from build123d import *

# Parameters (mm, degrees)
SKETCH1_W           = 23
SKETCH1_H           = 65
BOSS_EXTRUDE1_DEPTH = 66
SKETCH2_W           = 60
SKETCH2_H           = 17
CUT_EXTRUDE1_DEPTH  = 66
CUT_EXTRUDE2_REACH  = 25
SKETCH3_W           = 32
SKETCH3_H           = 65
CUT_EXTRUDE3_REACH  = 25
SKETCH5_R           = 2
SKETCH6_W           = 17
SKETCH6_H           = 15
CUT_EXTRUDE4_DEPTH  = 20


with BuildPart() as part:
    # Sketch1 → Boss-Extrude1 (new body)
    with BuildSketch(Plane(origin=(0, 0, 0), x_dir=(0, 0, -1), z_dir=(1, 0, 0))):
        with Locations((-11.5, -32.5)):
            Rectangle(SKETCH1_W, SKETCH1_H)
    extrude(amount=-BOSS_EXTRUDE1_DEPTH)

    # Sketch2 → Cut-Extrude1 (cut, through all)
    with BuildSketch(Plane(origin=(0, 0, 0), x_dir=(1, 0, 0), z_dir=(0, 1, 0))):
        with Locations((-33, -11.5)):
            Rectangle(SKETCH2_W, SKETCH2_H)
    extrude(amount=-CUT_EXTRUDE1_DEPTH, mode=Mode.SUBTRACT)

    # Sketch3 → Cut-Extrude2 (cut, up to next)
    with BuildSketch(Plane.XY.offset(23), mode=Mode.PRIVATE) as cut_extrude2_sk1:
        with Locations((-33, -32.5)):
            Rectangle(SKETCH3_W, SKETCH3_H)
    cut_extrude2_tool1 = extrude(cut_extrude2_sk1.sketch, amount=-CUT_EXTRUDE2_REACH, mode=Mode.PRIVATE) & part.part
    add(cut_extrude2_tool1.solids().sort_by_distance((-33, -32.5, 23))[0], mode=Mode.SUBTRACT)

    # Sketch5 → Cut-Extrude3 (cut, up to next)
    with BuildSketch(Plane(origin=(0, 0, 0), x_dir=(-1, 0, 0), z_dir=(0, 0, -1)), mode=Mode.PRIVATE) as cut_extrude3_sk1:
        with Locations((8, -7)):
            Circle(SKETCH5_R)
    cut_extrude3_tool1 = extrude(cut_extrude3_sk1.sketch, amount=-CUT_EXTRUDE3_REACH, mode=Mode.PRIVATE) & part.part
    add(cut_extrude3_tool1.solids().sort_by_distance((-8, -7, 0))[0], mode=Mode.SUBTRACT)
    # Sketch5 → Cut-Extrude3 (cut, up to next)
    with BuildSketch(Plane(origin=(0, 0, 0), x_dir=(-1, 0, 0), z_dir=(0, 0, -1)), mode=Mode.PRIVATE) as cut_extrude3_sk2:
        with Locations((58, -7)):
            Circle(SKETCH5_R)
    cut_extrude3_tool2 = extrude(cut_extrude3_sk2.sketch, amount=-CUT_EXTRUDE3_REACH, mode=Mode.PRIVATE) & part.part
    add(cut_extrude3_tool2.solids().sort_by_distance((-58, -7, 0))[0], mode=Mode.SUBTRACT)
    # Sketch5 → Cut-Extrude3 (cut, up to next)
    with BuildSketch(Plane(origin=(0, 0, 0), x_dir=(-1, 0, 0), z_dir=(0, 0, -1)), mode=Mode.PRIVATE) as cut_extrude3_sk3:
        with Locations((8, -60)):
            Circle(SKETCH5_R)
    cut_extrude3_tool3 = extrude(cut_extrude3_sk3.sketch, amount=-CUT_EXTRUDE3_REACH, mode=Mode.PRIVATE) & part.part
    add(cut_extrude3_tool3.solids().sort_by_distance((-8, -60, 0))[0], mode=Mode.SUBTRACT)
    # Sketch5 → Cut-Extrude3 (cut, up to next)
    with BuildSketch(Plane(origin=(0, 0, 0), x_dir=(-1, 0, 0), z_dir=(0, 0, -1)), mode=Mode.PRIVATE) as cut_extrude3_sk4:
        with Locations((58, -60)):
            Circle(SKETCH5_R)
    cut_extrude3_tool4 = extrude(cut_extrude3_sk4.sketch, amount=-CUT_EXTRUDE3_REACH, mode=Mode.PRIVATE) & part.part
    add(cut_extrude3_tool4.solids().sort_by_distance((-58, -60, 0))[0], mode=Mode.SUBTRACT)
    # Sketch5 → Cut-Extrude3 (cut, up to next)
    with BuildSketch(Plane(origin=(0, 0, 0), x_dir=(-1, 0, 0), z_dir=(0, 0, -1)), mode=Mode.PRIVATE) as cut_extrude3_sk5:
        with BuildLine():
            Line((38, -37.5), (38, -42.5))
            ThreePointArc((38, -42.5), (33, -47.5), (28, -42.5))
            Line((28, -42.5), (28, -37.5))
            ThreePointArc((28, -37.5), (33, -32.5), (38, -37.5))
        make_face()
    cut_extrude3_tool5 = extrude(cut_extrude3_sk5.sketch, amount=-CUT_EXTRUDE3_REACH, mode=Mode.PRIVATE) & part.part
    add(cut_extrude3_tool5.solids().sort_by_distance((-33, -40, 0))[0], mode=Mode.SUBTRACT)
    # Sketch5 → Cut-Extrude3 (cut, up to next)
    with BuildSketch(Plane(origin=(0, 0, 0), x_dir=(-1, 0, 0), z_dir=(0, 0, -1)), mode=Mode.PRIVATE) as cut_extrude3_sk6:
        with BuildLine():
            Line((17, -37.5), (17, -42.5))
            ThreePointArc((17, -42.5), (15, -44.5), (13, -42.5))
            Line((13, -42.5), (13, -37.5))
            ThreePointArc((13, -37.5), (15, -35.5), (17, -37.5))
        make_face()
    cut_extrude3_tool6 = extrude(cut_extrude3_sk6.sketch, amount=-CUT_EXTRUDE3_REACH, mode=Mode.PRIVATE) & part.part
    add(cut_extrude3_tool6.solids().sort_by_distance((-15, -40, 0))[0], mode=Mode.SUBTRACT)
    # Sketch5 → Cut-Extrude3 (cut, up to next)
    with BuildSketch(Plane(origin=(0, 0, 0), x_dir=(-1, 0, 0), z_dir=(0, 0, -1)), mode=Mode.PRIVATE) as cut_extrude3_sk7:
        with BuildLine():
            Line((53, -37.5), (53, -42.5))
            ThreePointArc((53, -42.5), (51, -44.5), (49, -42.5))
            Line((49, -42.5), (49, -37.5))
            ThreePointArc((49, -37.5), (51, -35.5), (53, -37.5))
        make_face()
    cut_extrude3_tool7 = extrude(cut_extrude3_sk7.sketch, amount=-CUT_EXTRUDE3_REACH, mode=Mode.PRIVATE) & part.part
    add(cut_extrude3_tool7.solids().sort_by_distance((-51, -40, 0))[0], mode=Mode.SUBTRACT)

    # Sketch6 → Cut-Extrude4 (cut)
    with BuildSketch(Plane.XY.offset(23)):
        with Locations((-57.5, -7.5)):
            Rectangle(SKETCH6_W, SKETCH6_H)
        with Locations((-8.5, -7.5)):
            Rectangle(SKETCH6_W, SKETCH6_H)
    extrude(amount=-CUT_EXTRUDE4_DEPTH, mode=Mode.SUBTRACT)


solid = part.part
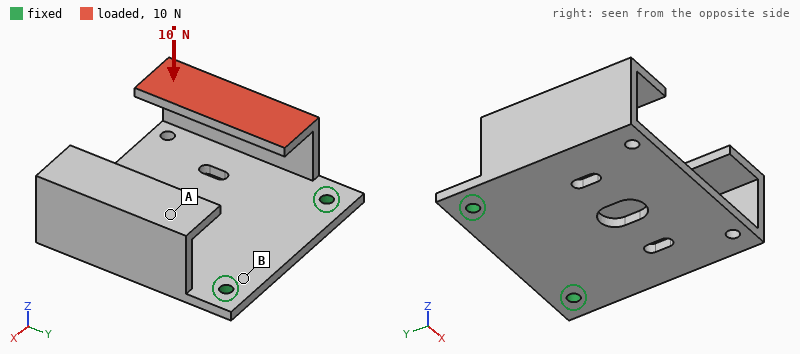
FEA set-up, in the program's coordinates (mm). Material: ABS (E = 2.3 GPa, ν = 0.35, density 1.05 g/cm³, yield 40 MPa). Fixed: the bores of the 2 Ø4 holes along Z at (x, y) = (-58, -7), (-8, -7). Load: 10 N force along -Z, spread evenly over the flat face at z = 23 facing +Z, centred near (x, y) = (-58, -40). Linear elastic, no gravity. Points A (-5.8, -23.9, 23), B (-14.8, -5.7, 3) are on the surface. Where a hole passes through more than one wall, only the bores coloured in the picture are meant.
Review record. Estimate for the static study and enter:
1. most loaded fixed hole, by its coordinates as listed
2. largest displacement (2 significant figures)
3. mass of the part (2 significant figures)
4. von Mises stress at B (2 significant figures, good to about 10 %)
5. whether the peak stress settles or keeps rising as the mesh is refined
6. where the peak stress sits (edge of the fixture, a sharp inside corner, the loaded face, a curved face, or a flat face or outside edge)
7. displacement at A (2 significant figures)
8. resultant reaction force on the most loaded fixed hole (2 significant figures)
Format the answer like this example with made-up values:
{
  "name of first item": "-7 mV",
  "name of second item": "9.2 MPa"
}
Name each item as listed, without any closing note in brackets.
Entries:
{
  "most loaded fixed hole, by its coordinates as listed": "(-58, -7)",
  "largest displacement": "1.1 mm",
  "mass of the part": "23 g",
  "von Mises stress at B": "1.8 MPa",
  "whether the peak stress settles or keeps rising as the mesh is refined": "keeps rising",
  "where the peak stress sits": "edge of the fixture",
  "displacement at A": "0.21 mm",
  "resultant reaction force on the most loaded fixed hole": "9.7 N"
}
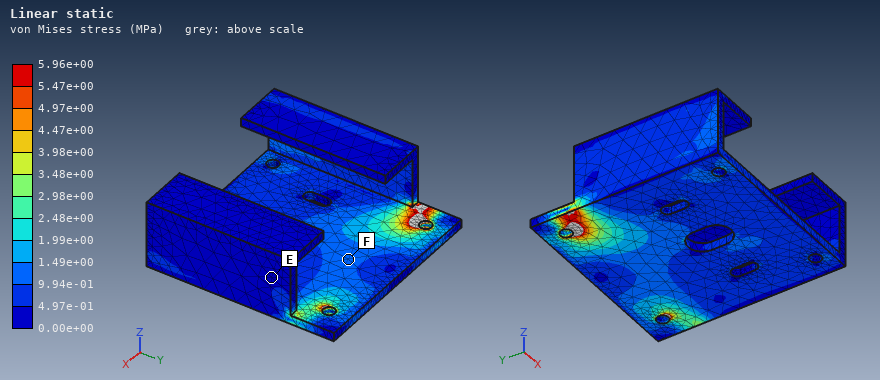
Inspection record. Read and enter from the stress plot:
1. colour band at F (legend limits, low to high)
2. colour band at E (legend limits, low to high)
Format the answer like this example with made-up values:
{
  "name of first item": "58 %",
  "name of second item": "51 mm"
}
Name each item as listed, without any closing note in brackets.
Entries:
{
  "colour band at F": "9.94e-01 to 1.49e+00 MPa",
  "colour band at E": "0.00e+00 to 4.97e-01 MPa"
}
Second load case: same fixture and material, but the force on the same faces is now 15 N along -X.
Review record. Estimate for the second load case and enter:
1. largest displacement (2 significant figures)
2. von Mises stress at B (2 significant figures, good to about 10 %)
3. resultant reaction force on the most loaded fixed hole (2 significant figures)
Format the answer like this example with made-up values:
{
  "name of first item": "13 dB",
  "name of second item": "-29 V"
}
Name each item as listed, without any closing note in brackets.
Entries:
{
  "largest displacement": "0.95 mm",
  "von Mises stress at B": "0.83 MPa",
  "resultant reaction force on the most loaded fixed hole": "13 N"
}
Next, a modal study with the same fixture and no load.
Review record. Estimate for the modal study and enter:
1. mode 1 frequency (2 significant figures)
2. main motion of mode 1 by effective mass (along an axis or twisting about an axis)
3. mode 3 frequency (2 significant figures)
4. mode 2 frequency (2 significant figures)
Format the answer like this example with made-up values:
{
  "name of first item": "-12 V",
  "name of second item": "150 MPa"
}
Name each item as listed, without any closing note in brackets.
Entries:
{
  "mode 1 frequency": "150 Hz",
  "main motion of mode 1 by effective mass": "along Z",
  "mode 3 frequency": "400 Hz",
  "mode 2 frequency": "240 Hz"
}
